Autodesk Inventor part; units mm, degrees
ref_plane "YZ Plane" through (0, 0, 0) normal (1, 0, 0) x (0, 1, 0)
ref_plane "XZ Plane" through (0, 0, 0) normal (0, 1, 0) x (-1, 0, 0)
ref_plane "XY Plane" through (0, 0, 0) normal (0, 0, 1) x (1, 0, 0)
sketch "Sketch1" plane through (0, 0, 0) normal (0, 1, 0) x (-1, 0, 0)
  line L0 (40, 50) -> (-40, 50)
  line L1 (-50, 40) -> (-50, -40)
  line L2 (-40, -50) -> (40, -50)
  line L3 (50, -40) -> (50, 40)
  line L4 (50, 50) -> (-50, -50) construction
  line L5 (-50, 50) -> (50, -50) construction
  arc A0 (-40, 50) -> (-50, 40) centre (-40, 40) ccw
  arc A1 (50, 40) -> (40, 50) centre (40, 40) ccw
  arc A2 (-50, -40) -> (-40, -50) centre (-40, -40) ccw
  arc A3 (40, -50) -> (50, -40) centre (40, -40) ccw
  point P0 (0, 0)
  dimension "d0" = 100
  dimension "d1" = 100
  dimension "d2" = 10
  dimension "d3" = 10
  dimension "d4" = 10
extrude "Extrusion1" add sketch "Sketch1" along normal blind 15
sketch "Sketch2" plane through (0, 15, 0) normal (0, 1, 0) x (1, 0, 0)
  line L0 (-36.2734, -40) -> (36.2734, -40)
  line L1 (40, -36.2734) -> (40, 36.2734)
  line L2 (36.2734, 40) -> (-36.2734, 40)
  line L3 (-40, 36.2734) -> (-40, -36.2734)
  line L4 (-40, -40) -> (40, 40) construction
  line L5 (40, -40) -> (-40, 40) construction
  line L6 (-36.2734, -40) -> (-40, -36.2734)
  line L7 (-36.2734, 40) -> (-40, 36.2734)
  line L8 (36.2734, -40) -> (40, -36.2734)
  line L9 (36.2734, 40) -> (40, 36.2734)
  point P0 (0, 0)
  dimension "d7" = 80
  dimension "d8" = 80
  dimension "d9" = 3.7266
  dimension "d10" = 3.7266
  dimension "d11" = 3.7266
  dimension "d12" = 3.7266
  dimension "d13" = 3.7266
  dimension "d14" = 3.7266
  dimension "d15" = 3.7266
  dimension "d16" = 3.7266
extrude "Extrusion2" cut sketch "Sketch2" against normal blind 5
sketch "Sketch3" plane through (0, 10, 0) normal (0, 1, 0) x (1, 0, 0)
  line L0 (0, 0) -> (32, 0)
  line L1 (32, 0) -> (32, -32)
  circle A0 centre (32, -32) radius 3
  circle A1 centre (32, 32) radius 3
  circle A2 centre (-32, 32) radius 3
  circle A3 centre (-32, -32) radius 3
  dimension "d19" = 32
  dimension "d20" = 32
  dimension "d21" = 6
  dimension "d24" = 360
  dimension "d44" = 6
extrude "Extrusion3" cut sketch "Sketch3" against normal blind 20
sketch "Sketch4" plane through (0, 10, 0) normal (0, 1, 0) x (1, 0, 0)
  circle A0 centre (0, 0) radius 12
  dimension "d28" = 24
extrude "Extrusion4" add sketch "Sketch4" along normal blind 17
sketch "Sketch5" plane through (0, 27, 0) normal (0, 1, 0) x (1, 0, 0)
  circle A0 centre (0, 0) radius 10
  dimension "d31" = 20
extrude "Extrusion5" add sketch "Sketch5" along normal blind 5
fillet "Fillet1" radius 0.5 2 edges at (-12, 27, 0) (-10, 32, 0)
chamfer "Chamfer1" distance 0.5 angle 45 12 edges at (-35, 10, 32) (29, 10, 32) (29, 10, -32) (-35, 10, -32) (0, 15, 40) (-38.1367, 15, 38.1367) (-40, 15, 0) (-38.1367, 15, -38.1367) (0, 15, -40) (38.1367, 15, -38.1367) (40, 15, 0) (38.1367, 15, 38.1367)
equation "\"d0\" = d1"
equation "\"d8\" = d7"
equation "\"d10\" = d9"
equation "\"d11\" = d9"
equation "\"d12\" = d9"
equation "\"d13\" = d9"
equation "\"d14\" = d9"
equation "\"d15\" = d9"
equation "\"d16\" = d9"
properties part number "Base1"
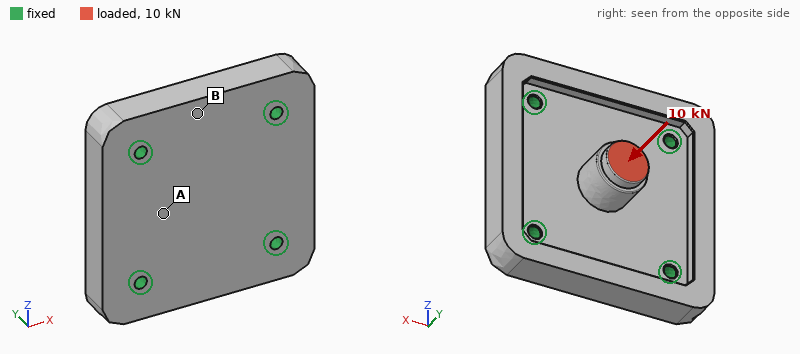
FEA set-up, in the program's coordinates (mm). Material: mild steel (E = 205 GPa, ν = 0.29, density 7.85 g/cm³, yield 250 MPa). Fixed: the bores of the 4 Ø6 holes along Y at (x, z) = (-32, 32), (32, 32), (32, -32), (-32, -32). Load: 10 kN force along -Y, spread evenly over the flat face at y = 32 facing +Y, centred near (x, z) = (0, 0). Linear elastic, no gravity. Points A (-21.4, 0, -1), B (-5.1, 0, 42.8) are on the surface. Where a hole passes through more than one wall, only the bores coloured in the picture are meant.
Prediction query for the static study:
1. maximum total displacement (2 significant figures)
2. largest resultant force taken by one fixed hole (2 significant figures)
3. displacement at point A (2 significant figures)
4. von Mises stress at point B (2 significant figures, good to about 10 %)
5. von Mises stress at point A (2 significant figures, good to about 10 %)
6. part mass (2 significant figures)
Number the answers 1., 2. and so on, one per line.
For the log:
1. 25 µm
2. 2.6 kN
3. 16 µm
4. 18 MPa
5. 35 MPa
6. 980 g
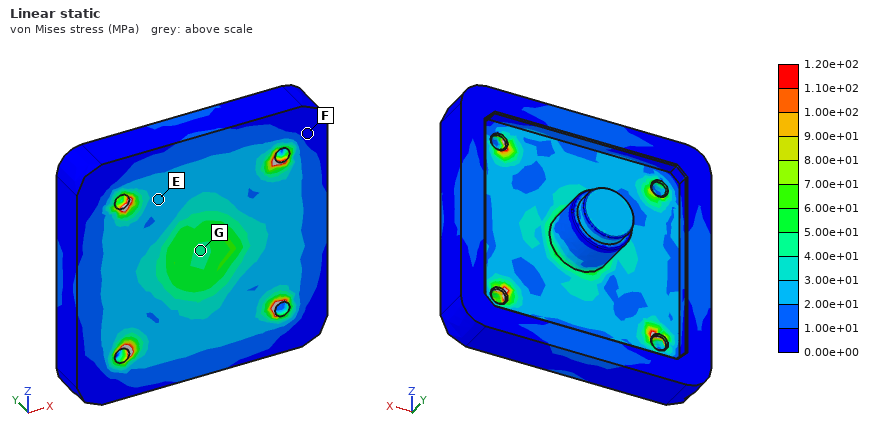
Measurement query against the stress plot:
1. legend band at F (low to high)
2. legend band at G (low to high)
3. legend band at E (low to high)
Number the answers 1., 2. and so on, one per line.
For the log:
1. 0.00e+00 to 1.00e+01 MPa
2. 4.00e+01 to 5.00e+01 MPa
3. 2.00e+01 to 3.00e+01 MPa
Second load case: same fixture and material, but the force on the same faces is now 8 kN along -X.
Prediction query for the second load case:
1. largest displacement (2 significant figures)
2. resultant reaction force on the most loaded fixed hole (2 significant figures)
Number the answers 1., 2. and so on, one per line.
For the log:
1. 47 µm
2. 2.9 kN
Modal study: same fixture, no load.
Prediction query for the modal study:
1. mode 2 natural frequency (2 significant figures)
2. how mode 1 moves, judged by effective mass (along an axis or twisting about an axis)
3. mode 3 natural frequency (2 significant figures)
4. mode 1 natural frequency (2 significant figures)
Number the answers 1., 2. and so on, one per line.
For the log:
1. 9300 Hz
2. along Y
3. 9700 Hz
4. 7100 Hz
